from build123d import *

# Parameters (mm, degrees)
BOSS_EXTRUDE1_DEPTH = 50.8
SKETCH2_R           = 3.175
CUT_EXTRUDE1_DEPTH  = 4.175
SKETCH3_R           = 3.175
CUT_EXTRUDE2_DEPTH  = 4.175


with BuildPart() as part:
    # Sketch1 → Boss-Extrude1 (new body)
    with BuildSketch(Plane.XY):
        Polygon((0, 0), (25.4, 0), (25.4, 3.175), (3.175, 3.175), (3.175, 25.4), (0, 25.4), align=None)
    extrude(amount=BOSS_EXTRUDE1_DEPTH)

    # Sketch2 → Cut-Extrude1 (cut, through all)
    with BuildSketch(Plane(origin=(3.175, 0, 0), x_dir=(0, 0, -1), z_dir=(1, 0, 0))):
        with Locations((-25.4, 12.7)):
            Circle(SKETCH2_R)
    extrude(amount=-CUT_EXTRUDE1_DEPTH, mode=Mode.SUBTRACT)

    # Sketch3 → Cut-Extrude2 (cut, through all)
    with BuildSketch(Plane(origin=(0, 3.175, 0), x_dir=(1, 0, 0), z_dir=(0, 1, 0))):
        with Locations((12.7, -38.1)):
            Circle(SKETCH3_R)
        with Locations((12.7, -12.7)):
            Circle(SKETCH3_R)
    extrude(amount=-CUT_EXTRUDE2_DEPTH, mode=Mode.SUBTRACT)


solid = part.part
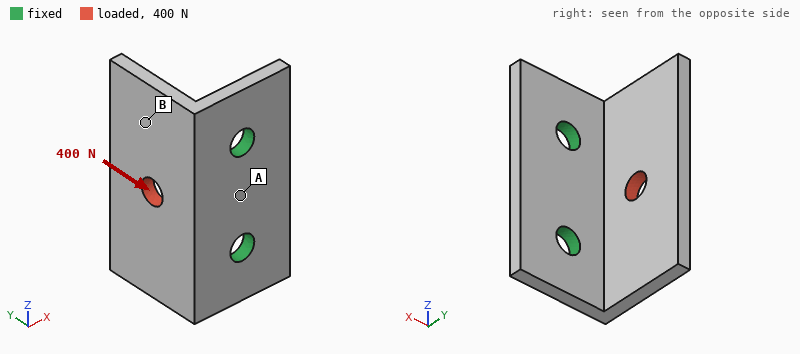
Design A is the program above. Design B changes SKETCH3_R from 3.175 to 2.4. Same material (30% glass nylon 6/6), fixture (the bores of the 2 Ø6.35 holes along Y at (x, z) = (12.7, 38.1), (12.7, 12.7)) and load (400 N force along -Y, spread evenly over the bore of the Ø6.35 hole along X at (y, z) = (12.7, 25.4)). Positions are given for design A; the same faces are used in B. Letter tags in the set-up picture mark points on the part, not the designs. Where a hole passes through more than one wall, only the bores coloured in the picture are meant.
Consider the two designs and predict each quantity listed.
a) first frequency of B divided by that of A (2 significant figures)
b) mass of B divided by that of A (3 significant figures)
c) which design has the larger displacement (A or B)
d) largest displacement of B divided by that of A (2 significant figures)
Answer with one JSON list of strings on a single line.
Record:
["0.95", "1.01", "B", "1.2"]
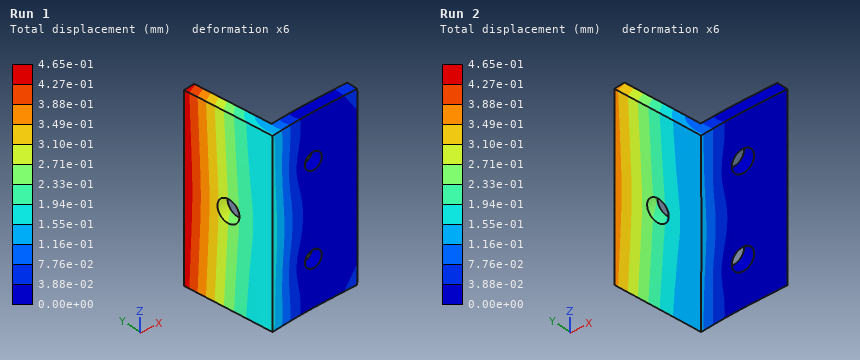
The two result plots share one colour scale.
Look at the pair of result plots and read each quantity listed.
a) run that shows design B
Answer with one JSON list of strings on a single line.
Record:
["Run 1"]
